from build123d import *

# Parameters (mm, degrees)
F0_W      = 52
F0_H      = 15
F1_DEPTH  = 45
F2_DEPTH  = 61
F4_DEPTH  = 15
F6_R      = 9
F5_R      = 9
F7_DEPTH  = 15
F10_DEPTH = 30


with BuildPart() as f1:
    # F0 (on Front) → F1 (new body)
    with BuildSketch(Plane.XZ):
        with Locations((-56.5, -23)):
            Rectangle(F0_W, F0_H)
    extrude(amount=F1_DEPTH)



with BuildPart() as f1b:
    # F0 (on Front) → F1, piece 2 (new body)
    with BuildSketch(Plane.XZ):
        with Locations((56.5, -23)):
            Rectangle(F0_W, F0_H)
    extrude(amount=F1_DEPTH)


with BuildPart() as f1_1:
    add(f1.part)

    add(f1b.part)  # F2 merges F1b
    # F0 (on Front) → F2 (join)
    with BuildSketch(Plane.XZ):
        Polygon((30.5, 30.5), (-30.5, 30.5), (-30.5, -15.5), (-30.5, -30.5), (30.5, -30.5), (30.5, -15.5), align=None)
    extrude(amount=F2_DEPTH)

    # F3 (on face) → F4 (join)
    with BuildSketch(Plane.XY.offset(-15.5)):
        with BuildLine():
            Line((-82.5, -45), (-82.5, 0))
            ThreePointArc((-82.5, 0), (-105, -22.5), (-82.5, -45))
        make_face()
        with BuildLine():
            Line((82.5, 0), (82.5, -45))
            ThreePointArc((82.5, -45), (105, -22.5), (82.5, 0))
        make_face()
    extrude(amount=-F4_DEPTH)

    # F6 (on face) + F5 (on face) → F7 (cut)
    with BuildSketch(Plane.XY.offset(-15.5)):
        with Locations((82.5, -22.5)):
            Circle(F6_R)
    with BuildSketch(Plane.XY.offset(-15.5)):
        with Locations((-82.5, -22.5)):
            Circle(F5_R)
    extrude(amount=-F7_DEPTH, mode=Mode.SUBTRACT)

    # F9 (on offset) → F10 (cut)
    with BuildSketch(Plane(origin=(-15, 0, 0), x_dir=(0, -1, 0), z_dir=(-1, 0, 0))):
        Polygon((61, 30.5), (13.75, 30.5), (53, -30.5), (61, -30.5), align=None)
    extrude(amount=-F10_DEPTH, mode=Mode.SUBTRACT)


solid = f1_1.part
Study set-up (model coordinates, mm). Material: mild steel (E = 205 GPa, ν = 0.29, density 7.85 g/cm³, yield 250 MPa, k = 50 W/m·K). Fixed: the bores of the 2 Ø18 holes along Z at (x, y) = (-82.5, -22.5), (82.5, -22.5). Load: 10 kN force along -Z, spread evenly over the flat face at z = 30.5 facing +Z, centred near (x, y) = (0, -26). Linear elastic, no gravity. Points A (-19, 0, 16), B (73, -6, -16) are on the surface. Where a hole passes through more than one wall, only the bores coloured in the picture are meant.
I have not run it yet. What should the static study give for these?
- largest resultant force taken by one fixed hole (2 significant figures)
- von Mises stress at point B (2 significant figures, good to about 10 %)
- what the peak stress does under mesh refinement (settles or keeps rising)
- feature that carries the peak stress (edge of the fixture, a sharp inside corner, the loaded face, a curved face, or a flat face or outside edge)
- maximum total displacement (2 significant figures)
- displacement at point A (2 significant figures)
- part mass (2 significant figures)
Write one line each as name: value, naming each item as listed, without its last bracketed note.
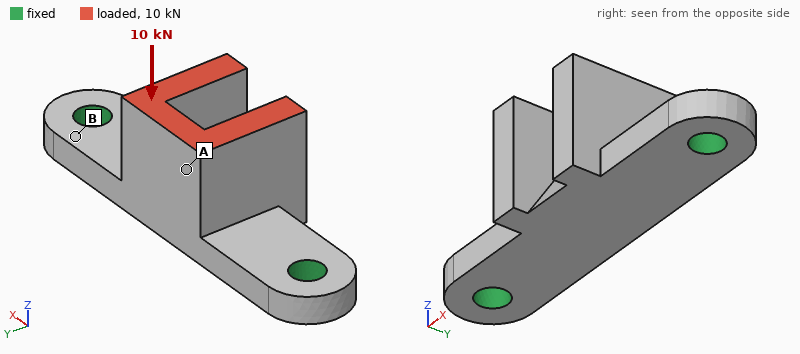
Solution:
largest resultant force taken by one fixed hole: 5.5 kN
von Mises stress at point B: 33 MPa
what the peak stress does under mesh refinement: keeps rising
feature that carries the peak stress: edge of the fixture
maximum total displacement: 45 µm
displacement at point A: 28 µm
part mass: 2.1 kg
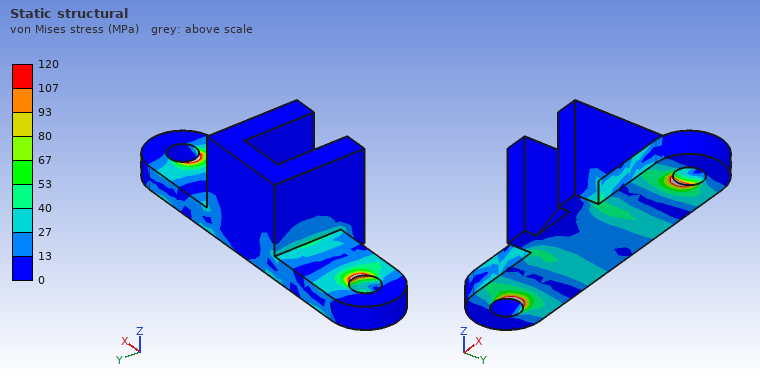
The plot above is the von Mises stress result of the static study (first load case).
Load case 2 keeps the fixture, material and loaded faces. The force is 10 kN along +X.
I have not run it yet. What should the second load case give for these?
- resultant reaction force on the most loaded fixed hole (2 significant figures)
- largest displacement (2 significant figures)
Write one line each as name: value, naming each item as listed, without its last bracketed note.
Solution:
resultant reaction force on the most loaded fixed hole: 6.9 kN
largest displacement: 53 µm
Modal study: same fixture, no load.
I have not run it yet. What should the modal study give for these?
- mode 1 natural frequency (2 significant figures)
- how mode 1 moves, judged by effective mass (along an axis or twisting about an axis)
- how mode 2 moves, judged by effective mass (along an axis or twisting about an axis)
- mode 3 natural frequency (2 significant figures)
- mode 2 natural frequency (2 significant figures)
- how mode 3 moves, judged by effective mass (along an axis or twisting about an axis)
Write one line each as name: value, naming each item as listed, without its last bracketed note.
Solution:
mode 1 natural frequency: 1500 Hz
how mode 1 moves, judged by effective mass: along Y
how mode 2 moves, judged by effective mass: along Z
mode 3 natural frequency: 3600 Hz
mode 2 natural frequency: 2300 Hz
how mode 3 moves, judged by effective mass: along X
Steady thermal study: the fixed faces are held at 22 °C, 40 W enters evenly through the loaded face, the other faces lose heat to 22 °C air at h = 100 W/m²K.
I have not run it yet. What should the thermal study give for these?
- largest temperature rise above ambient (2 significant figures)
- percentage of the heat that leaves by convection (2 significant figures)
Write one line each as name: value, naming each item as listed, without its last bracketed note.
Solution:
largest temperature rise above ambient: 20 K
percentage of the heat that leaves by convection: 76 %
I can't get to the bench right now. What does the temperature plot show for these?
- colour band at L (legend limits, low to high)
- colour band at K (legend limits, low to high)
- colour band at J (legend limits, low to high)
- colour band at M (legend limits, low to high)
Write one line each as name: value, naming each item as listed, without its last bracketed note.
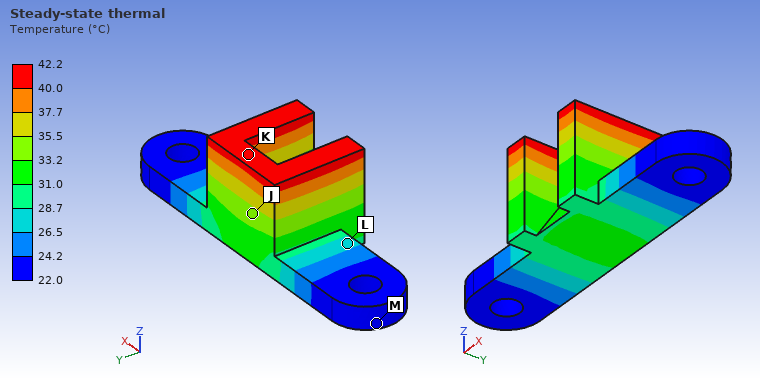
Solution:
colour band at L: 26.5 to 28.7 °C
colour band at K: 40.0 to 42.2 °C
colour band at J: 33.2 to 35.5 °C
colour band at M: 22.0 to 24.2 °C
